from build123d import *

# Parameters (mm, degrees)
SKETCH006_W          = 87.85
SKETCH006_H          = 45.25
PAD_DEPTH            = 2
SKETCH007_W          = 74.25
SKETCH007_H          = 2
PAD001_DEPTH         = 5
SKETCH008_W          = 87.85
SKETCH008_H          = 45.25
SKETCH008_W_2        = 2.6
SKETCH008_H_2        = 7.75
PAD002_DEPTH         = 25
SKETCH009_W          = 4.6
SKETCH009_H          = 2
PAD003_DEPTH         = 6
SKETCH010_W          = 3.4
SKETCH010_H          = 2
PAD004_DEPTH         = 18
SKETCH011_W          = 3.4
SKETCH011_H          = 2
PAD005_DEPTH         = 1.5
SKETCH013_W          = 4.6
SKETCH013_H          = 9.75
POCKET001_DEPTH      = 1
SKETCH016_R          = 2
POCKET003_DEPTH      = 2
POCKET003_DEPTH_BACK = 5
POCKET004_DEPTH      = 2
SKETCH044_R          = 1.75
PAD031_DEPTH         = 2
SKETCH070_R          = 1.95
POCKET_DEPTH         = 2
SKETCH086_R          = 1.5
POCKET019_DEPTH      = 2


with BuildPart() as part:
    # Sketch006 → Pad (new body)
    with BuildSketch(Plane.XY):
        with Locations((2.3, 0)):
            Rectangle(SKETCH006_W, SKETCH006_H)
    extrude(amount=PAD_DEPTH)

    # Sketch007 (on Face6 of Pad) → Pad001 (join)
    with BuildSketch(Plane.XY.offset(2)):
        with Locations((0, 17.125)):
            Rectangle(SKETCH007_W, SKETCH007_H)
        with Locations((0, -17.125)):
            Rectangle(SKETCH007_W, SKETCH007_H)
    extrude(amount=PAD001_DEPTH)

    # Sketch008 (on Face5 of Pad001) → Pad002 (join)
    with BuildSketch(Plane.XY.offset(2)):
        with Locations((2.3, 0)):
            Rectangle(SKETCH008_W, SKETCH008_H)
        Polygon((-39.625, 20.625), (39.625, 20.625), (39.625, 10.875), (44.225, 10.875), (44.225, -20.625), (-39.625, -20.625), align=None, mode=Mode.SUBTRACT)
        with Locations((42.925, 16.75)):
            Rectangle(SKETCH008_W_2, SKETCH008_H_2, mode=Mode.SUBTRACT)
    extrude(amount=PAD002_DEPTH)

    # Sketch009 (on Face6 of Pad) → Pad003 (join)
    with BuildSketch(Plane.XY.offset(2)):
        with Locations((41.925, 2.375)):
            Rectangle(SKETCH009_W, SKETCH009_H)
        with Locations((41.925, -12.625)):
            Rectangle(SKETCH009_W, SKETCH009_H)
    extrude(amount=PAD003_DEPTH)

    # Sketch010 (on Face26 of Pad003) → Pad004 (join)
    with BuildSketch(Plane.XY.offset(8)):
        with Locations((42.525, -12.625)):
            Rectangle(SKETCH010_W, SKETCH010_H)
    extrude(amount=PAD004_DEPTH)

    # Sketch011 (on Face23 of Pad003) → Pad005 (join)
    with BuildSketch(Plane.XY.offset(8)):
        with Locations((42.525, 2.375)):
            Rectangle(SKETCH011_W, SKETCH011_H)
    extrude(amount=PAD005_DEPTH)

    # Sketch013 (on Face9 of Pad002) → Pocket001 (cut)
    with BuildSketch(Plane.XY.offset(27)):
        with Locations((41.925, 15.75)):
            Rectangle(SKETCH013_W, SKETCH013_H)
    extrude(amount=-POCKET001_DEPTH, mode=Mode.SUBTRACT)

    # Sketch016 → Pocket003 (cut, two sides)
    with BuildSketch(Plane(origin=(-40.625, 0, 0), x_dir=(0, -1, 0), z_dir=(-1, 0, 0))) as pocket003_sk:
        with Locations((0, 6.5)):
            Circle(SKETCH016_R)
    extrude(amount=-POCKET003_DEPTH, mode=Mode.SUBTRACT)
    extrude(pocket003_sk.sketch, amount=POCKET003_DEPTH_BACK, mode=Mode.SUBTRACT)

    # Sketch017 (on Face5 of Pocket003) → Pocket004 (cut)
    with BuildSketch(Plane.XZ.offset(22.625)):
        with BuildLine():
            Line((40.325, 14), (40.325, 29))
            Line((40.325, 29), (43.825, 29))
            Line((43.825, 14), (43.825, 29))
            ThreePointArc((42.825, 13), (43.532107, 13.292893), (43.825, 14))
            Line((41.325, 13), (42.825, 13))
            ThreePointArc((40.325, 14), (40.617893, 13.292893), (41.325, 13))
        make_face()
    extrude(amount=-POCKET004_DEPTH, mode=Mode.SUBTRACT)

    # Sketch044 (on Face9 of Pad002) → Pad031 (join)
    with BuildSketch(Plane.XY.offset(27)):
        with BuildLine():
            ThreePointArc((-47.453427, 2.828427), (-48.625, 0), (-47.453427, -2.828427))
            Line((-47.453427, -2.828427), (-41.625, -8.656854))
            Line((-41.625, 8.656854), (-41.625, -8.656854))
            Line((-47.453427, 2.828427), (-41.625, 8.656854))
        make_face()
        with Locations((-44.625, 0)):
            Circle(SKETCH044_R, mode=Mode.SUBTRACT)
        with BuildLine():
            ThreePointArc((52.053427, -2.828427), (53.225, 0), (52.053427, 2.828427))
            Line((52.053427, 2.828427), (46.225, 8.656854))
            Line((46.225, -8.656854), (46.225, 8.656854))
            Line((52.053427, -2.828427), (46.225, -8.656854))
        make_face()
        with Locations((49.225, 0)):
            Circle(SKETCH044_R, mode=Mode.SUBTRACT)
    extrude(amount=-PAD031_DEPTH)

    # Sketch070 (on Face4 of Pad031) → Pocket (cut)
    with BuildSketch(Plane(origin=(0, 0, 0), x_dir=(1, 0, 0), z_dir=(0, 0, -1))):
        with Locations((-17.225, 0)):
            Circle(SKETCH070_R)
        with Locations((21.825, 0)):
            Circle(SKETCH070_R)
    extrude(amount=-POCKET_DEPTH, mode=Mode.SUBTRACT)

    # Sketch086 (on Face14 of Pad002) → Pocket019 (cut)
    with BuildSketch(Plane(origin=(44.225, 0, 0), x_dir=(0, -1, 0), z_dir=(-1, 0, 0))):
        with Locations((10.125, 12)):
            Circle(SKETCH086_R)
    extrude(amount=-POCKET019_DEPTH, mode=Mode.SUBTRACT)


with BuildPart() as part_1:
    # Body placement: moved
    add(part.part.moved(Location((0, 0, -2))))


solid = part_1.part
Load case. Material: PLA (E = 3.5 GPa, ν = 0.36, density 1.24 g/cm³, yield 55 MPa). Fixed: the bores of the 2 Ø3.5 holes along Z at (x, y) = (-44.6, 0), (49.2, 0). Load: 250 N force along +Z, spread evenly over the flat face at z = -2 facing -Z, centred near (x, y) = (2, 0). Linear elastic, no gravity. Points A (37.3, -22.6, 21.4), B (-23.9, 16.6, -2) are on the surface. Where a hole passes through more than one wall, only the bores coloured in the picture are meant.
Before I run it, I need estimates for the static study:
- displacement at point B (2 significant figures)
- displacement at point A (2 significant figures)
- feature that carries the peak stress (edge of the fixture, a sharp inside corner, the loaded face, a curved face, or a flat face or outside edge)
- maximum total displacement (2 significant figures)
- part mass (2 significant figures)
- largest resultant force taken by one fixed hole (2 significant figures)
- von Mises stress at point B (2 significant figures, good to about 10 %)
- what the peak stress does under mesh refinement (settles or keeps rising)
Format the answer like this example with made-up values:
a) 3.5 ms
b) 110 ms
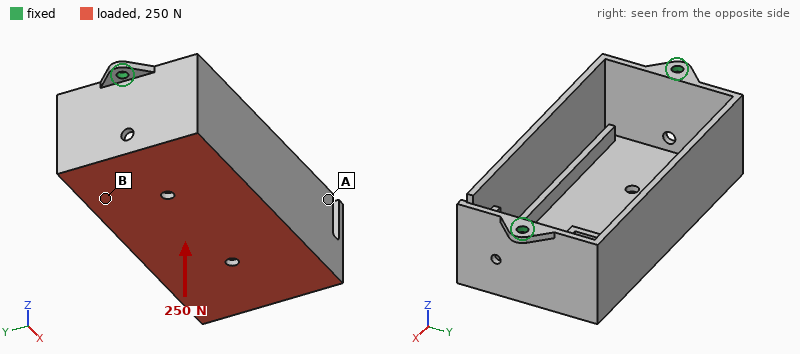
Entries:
a) 0.19 mm
b) 0.21 mm
c) edge of the fixture
d) 0.56 mm
e) 29 g
f) 130 N
g) 4.5 MPa
h) keeps rising
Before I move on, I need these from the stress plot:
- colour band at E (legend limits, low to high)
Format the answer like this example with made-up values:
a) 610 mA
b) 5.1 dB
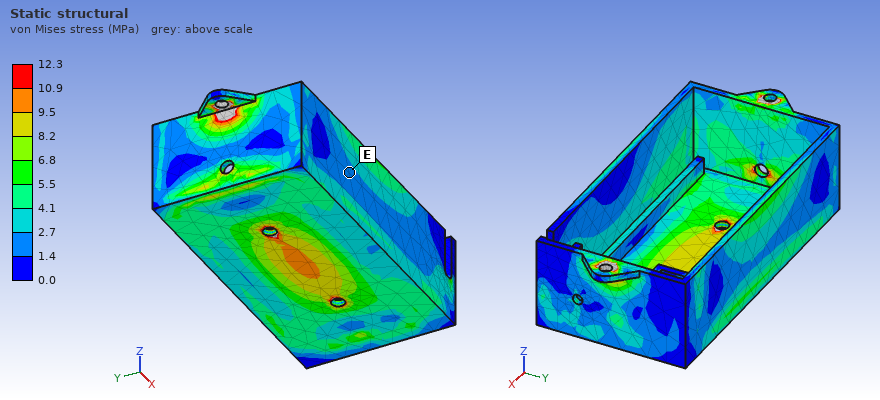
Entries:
a) 1.4 to 2.7 MPa
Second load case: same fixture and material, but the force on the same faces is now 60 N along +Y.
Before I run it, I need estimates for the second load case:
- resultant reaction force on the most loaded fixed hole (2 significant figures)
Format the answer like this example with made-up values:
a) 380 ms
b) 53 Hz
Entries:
a) 30 N
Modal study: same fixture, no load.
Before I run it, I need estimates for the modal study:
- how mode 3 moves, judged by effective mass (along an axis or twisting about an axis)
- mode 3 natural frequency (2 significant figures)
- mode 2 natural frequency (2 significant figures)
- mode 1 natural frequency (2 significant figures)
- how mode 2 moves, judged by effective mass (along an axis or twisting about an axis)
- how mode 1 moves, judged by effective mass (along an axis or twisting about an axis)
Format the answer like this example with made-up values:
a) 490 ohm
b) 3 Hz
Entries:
a) along X
b) 600 Hz
c) 450 Hz
d) 240 Hz
e) along X
f) along Y
